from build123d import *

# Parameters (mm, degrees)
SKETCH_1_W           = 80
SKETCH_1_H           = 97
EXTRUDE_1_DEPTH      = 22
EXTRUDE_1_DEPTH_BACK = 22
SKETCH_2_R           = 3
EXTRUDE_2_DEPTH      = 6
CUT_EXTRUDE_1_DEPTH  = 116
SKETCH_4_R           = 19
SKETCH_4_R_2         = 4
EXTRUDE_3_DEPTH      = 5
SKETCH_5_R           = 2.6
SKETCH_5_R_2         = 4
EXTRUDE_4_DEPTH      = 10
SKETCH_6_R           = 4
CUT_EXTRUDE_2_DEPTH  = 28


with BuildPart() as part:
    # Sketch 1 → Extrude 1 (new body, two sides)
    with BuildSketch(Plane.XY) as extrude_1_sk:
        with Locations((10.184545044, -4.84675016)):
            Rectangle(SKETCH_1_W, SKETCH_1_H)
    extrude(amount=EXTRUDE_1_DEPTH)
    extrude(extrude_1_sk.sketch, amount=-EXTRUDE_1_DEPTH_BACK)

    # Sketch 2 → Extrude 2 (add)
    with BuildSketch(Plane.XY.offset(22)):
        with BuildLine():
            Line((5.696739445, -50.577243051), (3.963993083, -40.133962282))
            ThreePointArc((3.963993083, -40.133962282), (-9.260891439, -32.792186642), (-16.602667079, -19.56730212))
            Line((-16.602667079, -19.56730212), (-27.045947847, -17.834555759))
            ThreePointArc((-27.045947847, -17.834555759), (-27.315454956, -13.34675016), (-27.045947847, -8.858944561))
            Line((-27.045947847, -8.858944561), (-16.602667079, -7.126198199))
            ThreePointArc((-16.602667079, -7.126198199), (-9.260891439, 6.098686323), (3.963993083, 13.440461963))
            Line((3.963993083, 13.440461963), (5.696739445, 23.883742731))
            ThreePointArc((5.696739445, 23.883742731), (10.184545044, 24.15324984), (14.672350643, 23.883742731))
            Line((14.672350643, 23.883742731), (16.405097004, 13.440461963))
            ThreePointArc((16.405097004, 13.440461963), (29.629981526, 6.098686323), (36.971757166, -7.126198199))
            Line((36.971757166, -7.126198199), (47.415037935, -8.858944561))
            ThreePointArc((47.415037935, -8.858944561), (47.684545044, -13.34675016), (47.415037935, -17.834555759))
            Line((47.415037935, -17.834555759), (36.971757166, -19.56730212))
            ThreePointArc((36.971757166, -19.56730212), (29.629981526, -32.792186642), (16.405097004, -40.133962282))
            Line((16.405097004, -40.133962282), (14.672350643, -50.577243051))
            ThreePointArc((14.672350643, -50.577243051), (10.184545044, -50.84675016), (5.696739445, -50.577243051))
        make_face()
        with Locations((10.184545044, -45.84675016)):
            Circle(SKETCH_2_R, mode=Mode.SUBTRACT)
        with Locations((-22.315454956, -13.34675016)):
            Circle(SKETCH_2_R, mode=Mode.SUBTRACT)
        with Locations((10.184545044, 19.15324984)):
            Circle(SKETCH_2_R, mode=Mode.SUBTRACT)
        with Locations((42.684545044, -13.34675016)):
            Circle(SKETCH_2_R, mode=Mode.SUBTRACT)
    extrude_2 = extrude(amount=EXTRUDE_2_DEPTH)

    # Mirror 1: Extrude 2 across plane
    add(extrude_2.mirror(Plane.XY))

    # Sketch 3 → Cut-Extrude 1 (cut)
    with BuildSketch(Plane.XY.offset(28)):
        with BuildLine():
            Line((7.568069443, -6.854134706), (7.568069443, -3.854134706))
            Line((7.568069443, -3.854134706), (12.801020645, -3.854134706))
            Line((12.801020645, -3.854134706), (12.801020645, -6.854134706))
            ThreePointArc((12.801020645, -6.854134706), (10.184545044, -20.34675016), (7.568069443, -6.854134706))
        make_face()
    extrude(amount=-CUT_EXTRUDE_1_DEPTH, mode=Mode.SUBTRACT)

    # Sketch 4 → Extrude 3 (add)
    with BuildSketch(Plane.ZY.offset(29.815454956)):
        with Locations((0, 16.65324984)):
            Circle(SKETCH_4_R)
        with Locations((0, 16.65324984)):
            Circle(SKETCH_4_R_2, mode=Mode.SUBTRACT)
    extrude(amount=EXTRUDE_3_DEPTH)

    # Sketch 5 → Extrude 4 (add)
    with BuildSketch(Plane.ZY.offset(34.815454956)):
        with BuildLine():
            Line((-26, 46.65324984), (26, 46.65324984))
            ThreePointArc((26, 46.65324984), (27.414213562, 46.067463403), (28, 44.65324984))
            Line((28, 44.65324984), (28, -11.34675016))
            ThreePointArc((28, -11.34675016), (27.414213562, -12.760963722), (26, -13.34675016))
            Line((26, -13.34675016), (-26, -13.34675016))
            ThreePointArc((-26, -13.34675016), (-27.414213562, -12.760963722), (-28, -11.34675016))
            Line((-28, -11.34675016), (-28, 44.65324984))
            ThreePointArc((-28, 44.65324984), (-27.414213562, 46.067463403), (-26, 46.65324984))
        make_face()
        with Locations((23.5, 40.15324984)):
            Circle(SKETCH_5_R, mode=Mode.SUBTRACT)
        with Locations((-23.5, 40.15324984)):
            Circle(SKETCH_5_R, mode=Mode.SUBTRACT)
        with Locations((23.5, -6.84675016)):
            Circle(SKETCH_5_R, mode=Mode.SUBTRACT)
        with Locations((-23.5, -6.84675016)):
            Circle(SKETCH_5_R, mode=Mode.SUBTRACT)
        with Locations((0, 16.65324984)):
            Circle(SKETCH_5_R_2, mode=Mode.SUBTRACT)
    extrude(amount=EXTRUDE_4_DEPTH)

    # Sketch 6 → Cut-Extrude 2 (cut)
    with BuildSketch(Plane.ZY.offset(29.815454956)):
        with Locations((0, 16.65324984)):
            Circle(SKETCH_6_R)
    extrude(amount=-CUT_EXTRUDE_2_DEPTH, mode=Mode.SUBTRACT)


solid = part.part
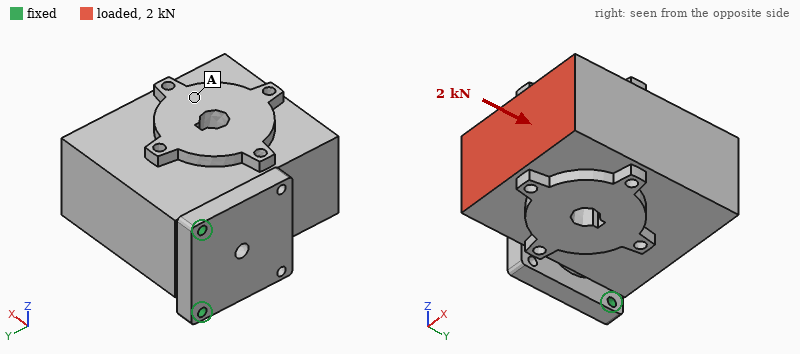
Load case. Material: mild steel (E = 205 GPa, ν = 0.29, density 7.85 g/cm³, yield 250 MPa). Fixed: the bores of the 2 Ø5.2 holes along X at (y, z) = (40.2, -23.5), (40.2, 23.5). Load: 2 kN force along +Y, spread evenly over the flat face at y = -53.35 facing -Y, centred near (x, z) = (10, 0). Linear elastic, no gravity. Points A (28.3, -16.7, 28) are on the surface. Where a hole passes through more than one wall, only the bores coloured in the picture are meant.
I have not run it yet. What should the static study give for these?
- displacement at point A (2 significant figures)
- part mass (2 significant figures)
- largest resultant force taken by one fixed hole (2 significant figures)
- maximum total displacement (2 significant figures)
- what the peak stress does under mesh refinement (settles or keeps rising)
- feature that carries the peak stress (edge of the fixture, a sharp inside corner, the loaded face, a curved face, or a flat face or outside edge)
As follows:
0.18 mm
3.1 kg
1.1 kN
0.26 mm
keeps rising
edge of the fixture
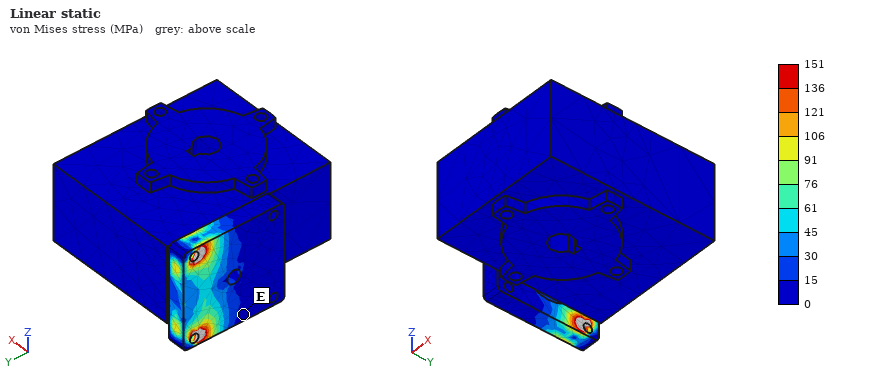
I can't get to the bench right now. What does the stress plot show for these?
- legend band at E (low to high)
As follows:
0 to 15 MPa
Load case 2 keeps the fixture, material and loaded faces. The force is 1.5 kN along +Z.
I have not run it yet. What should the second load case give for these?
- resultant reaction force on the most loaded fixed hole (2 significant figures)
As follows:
3.5 kN
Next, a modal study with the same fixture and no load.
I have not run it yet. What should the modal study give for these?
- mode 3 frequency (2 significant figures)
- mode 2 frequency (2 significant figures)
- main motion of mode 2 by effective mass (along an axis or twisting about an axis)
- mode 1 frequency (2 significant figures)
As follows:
2000 Hz
750 Hz
along Z
280 Hz
